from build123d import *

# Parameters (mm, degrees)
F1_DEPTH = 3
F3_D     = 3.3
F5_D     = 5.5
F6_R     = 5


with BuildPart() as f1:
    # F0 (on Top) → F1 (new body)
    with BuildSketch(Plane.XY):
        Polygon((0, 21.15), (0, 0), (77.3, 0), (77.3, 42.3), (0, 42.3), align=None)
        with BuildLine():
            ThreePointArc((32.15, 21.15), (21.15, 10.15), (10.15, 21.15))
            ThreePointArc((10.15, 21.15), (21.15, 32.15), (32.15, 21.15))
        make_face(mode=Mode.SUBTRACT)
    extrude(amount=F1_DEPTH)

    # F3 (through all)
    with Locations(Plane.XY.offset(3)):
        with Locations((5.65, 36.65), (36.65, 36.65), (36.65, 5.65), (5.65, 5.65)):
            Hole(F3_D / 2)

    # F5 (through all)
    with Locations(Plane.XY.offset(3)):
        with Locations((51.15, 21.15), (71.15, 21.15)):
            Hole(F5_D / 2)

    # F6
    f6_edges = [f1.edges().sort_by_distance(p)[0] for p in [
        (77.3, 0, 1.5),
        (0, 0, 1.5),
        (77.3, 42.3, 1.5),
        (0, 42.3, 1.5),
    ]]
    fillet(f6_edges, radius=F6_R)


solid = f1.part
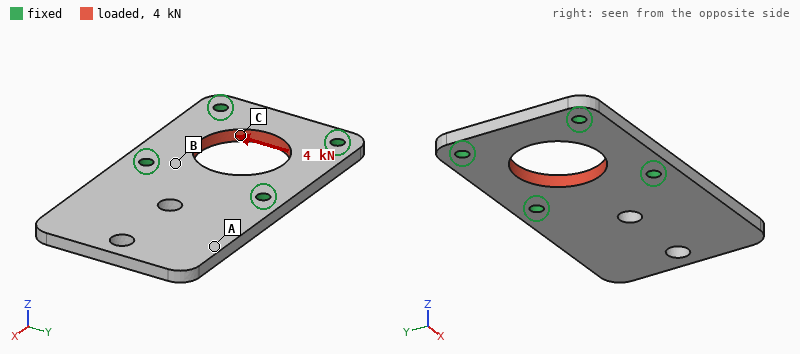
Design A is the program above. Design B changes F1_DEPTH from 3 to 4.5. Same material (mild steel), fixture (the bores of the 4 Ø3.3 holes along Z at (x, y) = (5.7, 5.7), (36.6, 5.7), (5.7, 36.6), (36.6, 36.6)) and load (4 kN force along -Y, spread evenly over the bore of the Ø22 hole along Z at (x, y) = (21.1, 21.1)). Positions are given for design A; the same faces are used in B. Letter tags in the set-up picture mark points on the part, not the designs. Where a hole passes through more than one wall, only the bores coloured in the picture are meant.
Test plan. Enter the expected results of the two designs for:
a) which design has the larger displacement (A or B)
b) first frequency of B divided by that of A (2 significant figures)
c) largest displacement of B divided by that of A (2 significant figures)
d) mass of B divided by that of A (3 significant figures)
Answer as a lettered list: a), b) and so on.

a) A
b) 1.5
c) 0.67
d) 1.50
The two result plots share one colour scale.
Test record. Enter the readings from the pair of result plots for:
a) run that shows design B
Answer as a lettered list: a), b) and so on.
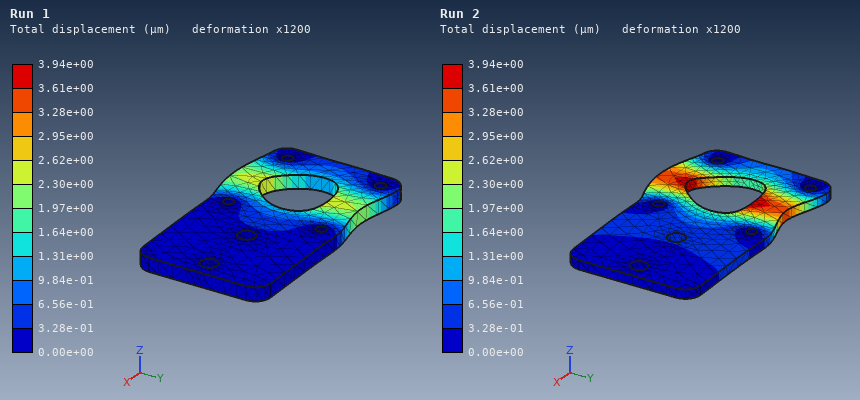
a) Run 1
